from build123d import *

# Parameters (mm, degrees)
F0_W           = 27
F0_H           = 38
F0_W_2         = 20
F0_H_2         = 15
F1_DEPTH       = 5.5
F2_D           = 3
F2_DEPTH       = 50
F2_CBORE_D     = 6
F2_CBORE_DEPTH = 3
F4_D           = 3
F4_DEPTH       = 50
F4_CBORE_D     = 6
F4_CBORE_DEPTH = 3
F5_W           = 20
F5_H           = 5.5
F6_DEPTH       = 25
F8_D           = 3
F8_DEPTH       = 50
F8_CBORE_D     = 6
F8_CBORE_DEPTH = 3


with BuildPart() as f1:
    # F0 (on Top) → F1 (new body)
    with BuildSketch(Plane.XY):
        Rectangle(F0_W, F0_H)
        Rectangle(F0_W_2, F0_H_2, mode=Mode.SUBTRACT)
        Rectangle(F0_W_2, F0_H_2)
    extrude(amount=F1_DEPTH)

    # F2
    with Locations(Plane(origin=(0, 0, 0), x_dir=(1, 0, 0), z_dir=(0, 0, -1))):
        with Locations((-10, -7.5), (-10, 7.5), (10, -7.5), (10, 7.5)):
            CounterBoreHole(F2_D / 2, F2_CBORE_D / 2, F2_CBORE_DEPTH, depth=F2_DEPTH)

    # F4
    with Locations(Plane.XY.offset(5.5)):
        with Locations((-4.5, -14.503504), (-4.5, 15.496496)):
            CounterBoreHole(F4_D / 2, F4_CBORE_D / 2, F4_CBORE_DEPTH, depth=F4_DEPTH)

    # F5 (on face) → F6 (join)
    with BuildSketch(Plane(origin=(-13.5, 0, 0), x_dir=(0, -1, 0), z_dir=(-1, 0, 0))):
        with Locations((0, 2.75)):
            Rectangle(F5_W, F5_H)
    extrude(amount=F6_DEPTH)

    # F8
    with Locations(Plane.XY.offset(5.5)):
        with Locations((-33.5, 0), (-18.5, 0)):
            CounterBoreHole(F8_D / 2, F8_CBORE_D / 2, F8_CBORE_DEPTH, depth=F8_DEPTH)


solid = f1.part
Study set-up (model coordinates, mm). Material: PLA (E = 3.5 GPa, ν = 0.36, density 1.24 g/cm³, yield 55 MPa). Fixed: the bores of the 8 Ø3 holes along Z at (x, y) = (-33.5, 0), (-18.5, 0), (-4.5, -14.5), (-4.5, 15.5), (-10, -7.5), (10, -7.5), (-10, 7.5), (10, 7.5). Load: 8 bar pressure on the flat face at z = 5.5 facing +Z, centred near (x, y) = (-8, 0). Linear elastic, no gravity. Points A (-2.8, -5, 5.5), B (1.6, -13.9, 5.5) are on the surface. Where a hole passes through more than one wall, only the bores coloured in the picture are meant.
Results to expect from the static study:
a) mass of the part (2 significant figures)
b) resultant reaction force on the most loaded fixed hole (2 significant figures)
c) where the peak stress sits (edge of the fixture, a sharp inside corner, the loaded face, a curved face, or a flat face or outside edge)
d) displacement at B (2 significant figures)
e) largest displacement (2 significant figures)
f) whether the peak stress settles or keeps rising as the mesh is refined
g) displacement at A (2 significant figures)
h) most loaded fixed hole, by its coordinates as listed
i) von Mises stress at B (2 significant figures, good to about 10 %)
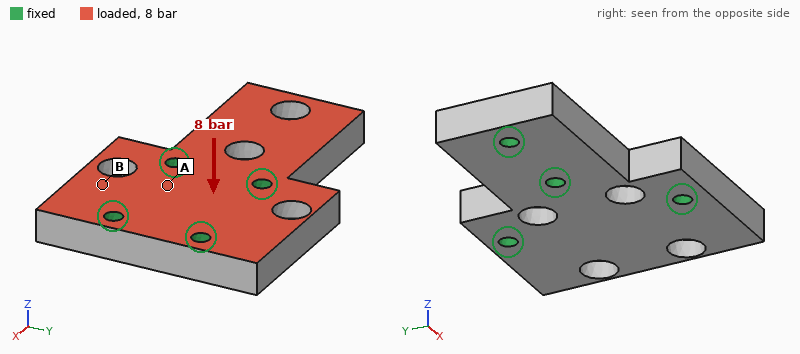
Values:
9.4 g
180 N
edge of the fixture
21 µm
56 µm
keeps rising
15 µm
(-33.5, 0)
4.4 MPa
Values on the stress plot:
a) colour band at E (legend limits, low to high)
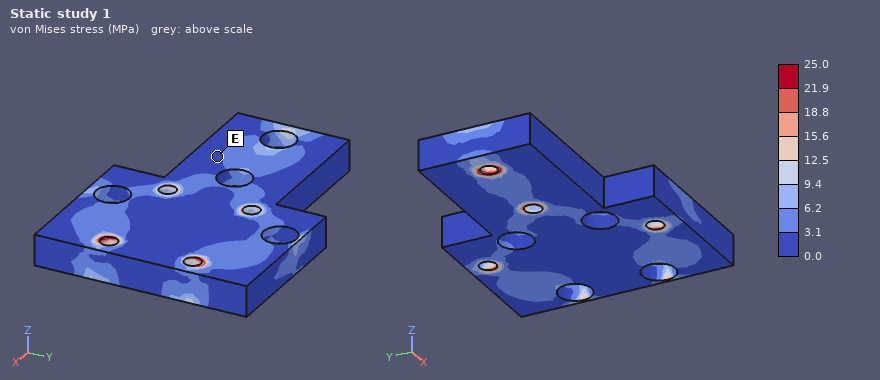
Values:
0.0 to 3.1 MPa
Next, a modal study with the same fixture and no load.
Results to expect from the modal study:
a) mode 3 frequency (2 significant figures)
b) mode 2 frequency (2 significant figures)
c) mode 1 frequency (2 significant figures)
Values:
9200 Hz
9000 Hz
6700 Hz
